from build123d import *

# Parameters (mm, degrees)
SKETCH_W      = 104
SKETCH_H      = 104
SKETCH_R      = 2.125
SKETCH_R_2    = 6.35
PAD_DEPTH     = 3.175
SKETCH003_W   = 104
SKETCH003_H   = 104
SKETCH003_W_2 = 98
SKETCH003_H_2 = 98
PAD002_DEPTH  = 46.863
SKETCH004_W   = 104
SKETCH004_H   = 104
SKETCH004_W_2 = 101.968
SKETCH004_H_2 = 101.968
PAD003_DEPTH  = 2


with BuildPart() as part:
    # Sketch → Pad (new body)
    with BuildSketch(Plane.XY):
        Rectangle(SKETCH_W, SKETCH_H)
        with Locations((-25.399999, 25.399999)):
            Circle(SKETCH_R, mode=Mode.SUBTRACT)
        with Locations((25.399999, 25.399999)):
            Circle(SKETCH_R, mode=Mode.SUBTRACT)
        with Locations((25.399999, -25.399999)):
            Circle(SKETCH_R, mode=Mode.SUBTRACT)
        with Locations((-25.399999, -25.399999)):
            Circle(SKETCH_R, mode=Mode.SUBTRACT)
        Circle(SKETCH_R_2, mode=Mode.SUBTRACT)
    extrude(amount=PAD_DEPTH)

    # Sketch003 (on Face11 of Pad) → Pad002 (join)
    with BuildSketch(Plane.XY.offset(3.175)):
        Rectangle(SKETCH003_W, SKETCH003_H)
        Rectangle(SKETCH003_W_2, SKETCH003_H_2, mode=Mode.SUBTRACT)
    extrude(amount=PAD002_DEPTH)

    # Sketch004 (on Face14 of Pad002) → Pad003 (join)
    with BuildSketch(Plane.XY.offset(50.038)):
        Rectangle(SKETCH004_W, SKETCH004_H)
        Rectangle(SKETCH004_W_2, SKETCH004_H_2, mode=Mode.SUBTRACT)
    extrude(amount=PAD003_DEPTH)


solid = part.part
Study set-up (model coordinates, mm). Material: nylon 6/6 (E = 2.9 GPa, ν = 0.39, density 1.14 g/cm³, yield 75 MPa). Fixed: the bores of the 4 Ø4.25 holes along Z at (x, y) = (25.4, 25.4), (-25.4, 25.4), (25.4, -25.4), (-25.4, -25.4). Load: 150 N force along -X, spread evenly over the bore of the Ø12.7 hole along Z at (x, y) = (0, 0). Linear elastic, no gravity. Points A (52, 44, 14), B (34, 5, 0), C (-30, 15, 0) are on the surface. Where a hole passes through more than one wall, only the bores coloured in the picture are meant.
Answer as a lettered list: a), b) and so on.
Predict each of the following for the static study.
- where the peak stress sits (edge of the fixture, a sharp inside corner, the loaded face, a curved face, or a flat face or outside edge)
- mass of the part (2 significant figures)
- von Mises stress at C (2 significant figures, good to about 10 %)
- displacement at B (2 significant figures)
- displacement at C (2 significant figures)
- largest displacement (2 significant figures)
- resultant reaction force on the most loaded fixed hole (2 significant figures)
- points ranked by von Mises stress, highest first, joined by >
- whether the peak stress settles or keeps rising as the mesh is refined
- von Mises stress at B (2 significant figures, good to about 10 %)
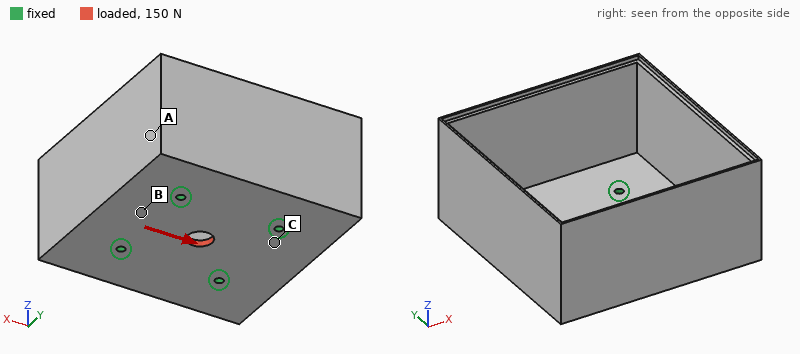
a) edge of the fixture
b) 100 g
c) 0.36 MPa
d) 4.5 µm
e) 3.4 µm
f) 10 µm
g) 39 N
h) C > B > A
i) keeps rising
j) 0.26 MPa
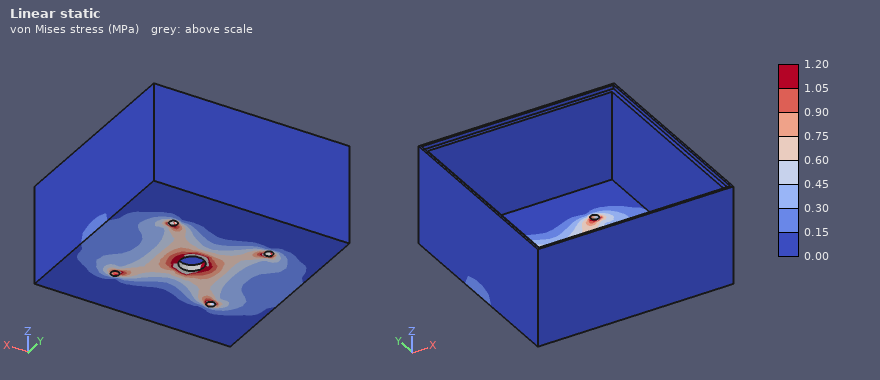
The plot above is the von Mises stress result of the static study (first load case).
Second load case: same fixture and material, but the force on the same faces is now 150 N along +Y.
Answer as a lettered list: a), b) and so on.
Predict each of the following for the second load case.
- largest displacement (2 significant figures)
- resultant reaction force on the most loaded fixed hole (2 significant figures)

a) 10 µm
b) 39 N
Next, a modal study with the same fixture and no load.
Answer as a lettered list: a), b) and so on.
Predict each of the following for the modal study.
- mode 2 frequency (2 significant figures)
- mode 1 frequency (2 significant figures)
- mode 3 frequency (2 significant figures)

a) 350 Hz
b) 310 Hz
c) 350 Hz
